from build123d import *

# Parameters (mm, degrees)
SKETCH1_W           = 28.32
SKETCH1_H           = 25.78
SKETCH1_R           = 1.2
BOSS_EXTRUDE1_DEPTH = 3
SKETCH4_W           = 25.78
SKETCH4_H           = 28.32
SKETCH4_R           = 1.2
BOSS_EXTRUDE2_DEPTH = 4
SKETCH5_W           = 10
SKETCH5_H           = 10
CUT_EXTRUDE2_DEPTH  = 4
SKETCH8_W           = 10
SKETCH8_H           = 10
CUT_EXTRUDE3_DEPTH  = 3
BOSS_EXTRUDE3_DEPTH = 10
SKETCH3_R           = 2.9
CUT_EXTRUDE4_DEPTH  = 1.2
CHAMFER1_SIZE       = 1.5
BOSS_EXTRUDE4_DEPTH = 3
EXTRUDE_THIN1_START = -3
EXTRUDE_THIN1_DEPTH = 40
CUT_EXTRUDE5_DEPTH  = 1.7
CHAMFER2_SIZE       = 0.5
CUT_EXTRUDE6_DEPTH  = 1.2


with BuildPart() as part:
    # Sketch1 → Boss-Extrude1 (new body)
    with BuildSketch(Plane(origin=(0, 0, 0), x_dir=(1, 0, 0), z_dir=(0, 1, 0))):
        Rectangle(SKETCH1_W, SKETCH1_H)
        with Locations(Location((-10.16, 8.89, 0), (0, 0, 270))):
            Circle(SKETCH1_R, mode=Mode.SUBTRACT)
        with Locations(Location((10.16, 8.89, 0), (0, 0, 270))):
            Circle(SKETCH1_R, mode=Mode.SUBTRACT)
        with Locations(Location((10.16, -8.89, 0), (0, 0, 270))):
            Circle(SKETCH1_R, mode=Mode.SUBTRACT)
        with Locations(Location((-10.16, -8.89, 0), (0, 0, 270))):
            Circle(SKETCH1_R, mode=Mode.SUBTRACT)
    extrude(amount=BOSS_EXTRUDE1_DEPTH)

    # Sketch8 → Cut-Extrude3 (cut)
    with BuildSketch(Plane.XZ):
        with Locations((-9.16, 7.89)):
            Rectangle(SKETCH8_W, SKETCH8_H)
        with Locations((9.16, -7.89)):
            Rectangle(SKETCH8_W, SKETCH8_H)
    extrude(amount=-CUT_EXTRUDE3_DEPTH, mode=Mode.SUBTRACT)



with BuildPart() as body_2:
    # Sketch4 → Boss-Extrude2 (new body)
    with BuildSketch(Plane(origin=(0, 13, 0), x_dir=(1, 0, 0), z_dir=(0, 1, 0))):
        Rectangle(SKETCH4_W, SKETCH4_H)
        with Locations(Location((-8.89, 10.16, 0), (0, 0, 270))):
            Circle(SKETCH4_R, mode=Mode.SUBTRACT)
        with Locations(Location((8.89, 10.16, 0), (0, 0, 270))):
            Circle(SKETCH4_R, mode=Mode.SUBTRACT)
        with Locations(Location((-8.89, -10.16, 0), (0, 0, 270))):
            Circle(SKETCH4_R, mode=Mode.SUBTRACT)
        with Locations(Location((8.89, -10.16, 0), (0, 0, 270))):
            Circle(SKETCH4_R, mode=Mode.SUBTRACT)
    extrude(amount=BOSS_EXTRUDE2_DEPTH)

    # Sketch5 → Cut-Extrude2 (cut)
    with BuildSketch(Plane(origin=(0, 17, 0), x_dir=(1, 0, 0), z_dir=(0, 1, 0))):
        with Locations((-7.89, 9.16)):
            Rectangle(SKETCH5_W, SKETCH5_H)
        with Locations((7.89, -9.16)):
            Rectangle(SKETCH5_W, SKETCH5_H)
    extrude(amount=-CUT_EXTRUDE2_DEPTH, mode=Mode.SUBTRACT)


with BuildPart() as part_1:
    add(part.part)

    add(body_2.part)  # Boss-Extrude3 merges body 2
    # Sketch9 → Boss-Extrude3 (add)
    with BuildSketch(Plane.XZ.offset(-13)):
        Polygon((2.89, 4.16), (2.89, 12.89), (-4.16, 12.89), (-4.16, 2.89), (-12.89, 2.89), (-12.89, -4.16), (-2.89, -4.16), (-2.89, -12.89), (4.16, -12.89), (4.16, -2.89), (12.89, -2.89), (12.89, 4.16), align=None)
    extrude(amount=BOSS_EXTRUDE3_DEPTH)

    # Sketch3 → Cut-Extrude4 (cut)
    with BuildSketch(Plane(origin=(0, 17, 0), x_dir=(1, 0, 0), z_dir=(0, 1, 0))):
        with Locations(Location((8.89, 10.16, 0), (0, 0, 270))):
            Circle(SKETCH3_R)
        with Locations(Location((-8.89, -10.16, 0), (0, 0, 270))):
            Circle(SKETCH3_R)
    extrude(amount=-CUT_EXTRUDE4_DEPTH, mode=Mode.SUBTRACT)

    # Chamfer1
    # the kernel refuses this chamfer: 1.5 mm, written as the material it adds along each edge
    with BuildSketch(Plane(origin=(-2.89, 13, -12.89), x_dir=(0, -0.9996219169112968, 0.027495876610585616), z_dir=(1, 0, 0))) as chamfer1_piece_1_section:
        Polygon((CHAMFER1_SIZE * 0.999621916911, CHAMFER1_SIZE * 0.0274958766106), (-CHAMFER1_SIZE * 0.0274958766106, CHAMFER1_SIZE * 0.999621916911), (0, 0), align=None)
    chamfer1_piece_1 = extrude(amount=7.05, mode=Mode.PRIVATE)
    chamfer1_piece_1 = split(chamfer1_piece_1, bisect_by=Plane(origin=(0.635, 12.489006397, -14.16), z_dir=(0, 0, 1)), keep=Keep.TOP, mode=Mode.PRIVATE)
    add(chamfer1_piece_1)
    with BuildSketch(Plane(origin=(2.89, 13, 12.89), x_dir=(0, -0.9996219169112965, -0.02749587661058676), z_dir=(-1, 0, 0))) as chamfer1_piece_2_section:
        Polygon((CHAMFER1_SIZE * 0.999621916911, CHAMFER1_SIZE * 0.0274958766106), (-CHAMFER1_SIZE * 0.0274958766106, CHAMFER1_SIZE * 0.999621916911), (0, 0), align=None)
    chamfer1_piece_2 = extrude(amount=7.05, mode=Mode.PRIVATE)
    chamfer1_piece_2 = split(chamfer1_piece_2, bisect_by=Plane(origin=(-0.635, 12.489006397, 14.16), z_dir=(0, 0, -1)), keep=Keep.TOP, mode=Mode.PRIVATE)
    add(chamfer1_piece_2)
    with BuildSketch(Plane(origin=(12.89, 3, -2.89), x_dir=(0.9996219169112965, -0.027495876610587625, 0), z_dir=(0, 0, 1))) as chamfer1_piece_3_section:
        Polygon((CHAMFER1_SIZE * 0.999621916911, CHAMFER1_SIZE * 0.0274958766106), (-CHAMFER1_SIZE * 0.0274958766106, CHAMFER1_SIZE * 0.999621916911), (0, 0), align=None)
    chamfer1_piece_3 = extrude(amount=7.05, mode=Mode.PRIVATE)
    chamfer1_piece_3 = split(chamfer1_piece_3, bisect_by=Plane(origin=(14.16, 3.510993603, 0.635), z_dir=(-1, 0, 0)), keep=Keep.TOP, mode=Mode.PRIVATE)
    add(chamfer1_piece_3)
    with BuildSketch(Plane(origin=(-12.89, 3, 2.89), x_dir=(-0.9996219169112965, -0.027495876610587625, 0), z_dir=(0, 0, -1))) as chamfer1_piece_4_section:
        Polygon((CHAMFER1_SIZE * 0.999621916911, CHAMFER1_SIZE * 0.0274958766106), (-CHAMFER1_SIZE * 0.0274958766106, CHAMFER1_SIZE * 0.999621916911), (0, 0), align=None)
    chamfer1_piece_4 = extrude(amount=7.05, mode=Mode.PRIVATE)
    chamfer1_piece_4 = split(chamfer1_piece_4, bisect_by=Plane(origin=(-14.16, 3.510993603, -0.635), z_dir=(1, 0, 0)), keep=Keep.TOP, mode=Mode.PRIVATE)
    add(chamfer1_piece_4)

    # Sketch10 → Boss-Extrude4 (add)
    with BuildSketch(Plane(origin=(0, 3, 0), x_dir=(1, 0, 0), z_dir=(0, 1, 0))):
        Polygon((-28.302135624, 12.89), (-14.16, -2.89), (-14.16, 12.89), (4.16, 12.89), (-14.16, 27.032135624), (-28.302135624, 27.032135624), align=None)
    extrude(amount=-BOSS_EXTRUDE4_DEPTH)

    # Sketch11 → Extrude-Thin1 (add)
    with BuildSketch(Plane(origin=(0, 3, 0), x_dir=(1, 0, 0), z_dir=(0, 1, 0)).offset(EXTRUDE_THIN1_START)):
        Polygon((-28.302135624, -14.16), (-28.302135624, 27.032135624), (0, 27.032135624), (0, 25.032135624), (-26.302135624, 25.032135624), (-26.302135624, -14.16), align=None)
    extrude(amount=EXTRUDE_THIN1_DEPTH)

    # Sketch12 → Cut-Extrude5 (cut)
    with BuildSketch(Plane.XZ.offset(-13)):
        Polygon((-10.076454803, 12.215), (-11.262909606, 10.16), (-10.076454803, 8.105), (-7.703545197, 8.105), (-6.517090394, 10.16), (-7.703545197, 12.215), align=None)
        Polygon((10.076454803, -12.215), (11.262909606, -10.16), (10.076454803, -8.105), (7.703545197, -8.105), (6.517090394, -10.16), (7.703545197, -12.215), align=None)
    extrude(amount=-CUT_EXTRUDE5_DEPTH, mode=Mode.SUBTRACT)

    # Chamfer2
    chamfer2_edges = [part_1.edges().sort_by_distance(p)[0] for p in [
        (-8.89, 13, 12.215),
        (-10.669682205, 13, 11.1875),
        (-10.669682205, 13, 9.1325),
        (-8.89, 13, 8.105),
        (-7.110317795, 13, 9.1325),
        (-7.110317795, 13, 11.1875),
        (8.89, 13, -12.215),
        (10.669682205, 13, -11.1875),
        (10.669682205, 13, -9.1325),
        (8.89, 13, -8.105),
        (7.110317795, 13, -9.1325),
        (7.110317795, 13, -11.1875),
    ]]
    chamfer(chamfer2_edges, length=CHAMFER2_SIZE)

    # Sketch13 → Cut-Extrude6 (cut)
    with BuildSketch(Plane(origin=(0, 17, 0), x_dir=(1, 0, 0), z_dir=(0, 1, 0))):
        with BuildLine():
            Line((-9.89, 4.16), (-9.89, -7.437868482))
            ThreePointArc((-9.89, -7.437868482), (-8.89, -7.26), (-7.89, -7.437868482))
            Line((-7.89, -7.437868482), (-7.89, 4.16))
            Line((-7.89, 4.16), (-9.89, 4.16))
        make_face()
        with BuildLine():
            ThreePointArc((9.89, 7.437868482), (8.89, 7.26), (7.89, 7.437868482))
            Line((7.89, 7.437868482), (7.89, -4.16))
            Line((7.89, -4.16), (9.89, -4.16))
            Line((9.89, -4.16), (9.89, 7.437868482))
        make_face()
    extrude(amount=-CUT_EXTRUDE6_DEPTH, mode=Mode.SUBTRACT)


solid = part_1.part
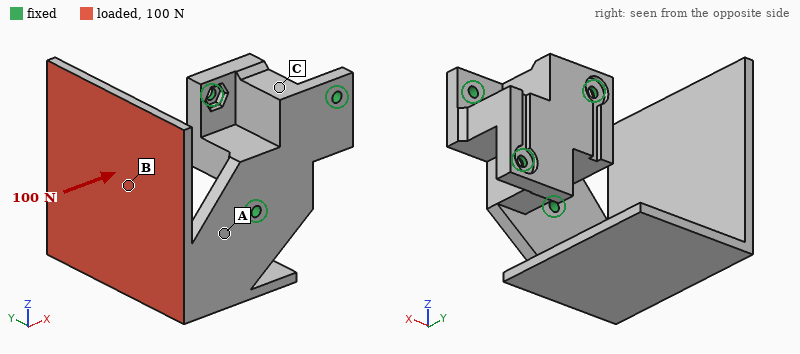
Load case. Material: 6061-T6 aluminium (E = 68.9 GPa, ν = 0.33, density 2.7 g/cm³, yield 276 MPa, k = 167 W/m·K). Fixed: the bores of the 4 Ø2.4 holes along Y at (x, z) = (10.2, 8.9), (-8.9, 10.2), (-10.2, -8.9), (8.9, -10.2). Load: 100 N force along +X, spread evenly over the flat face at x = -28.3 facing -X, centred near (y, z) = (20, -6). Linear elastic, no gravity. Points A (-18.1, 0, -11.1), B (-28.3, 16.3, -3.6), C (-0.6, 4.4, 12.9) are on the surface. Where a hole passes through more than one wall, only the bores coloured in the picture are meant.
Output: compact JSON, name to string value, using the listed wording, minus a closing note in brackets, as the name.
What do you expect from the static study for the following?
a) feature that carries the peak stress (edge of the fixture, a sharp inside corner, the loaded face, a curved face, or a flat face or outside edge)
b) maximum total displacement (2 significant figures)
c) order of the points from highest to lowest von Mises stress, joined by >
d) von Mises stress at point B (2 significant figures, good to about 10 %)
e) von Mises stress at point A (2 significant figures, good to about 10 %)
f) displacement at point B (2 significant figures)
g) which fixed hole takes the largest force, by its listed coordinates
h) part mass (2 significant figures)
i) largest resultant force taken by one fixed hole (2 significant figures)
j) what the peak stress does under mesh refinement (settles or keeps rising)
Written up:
{"feature that carries the peak stress": "edge of the fixture", "maximum total displacement": "0.70 mm", "order of the points from highest to lowest von Mises stress, joined by >": "A > B > C", "von Mises stress at point B": "19 MPa", "von Mises stress at point A": "40 MPa", "displacement at point B": "0.23 mm", "which fixed hole takes the largest force, by its listed coordinates": "(-10.2, -8.9)", "part mass": "36 g", "largest resultant force taken by one fixed hole": "110 N", "what the peak stress does under mesh refinement": "keeps rising"}
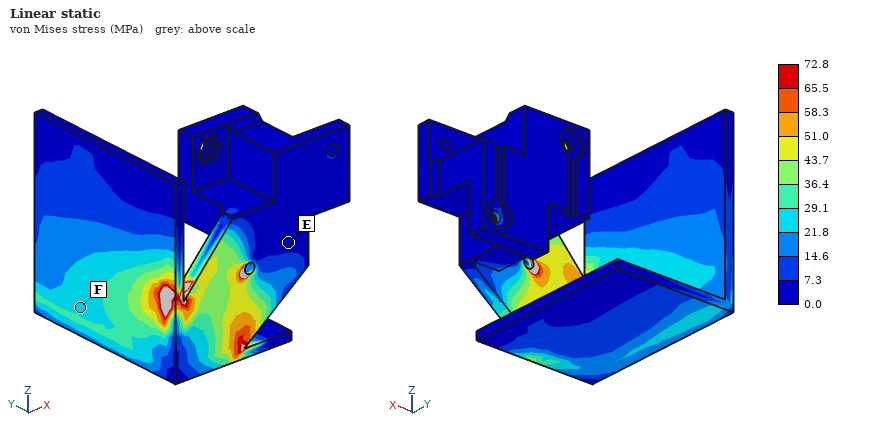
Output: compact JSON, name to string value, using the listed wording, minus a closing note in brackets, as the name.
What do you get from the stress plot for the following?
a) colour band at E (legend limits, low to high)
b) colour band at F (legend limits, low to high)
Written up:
{"colour band at E": "0.0 to 7.3 MPa", "colour band at F": "21.8 to 29.1 MPa"}
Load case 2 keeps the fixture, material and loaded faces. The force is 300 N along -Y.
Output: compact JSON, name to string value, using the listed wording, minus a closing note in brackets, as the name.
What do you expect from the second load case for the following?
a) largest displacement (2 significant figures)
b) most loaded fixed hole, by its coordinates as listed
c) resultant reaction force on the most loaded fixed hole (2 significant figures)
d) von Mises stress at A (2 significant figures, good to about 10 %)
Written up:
{"largest displacement": "0.62 mm", "most loaded fixed hole, by its coordinates as listed": "(-10.2, -8.9)", "resultant reaction force on the most loaded fixed hole": "380 N", "von Mises stress at A": "93 MPa"}
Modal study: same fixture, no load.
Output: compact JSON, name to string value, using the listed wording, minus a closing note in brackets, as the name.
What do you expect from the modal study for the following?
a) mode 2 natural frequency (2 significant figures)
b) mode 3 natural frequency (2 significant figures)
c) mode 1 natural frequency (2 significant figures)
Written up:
{"mode 2 natural frequency": "860 Hz", "mode 3 natural frequency": "1600 Hz", "mode 1 natural frequency": "740 Hz"}
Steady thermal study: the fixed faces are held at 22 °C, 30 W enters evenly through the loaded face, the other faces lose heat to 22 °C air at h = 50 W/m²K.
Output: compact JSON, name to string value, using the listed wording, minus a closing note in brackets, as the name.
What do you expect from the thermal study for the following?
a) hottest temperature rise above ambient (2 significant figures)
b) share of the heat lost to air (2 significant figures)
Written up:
{"hottest temperature rise above ambient": "73 K", "share of the heat lost to air": "38 %"}
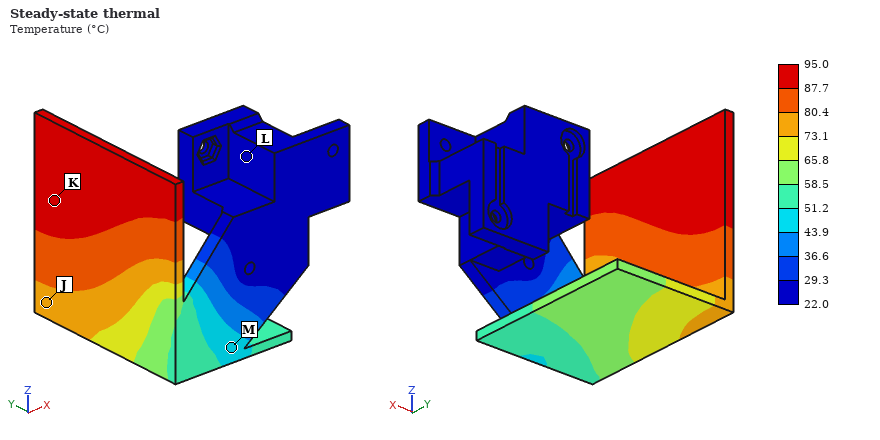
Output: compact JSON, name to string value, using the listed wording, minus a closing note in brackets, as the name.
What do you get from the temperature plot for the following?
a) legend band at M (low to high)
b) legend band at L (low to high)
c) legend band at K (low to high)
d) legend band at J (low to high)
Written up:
{"legend band at M": "43.9 to 51.2 °C", "legend band at L": "22.0 to 29.3 °C", "legend band at K": "87.7 to 95.0 °C", "legend band at J": "73.1 to 80.4 °C"}
